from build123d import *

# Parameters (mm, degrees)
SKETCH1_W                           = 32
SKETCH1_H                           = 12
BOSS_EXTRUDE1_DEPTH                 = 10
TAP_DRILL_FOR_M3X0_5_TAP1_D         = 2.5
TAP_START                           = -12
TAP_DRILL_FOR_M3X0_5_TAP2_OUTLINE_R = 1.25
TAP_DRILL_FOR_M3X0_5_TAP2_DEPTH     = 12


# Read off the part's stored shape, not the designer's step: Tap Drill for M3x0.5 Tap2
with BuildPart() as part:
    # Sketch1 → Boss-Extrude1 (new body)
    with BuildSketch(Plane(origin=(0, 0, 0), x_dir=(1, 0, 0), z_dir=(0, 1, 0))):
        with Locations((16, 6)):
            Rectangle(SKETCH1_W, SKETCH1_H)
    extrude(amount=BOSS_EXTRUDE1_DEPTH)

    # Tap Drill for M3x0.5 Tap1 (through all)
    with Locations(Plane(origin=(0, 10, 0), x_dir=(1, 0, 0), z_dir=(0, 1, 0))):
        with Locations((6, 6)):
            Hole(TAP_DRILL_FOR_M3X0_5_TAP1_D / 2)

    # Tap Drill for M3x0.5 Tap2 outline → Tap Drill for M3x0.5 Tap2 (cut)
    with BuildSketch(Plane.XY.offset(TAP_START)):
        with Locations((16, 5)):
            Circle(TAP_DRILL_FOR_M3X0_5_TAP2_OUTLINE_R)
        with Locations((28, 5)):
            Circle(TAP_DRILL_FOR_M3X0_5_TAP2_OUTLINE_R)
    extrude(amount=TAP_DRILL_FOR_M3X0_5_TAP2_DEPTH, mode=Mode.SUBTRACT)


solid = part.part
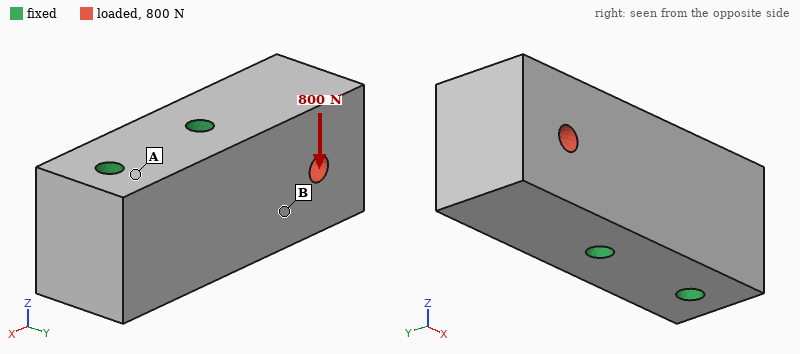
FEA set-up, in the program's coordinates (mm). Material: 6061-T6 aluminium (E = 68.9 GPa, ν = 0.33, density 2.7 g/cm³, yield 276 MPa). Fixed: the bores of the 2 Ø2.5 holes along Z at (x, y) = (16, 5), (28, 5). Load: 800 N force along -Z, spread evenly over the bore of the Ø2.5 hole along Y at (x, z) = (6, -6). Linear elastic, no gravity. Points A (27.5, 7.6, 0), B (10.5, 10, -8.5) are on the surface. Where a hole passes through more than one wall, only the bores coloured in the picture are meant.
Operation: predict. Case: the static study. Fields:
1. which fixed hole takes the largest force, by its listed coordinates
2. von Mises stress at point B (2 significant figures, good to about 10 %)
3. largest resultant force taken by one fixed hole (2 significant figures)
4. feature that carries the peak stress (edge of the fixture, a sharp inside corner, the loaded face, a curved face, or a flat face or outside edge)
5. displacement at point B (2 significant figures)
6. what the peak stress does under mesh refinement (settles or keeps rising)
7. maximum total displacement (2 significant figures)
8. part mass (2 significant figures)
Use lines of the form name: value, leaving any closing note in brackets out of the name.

which fixed hole takes the largest force, by its listed coordinates: (16, 5)
von Mises stress at point B: 14 MPa
largest resultant force taken by one fixed hole: 870 N
feature that carries the peak stress: edge of the fixture
displacement at point B: 2.9 µm
what the peak stress does under mesh refinement: keeps rising
maximum total displacement: 9.6 µm
part mass: 9.9 g
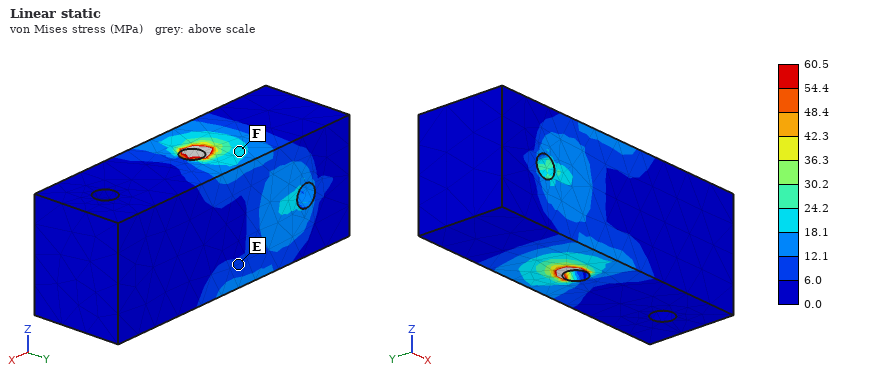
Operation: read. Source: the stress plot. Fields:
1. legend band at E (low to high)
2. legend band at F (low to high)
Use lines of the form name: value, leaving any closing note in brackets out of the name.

legend band at E: 6.0 to 12.1 MPa
legend band at F: 18.1 to 24.2 MPa
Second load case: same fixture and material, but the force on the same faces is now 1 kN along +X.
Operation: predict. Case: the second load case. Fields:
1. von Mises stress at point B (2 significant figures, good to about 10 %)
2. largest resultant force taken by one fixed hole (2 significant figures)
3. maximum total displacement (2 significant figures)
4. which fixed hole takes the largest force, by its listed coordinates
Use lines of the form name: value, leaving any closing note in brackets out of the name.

von Mises stress at point B: 8.4 MPa
largest resultant force taken by one fixed hole: 880 N
maximum total displacement: 2.0 µm
which fixed hole takes the largest force, by its listed coordinates: (16, 5)
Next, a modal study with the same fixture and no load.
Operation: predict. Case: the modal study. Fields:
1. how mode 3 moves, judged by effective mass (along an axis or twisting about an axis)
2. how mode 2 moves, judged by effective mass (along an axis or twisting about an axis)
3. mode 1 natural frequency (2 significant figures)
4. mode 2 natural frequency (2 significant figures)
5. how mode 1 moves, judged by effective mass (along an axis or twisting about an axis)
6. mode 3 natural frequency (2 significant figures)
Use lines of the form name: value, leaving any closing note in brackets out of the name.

how mode 3 moves, judged by effective mass: twisting about X
how mode 2 moves, judged by effective mass: along Z
mode 1 natural frequency: 20 kHz
mode 2 natural frequency: 27 kHz
how mode 1 moves, judged by effective mass: along Y
mode 3 natural frequency: 43 kHz
